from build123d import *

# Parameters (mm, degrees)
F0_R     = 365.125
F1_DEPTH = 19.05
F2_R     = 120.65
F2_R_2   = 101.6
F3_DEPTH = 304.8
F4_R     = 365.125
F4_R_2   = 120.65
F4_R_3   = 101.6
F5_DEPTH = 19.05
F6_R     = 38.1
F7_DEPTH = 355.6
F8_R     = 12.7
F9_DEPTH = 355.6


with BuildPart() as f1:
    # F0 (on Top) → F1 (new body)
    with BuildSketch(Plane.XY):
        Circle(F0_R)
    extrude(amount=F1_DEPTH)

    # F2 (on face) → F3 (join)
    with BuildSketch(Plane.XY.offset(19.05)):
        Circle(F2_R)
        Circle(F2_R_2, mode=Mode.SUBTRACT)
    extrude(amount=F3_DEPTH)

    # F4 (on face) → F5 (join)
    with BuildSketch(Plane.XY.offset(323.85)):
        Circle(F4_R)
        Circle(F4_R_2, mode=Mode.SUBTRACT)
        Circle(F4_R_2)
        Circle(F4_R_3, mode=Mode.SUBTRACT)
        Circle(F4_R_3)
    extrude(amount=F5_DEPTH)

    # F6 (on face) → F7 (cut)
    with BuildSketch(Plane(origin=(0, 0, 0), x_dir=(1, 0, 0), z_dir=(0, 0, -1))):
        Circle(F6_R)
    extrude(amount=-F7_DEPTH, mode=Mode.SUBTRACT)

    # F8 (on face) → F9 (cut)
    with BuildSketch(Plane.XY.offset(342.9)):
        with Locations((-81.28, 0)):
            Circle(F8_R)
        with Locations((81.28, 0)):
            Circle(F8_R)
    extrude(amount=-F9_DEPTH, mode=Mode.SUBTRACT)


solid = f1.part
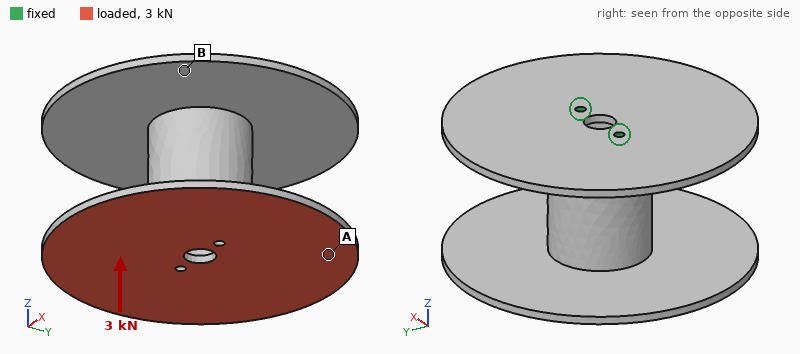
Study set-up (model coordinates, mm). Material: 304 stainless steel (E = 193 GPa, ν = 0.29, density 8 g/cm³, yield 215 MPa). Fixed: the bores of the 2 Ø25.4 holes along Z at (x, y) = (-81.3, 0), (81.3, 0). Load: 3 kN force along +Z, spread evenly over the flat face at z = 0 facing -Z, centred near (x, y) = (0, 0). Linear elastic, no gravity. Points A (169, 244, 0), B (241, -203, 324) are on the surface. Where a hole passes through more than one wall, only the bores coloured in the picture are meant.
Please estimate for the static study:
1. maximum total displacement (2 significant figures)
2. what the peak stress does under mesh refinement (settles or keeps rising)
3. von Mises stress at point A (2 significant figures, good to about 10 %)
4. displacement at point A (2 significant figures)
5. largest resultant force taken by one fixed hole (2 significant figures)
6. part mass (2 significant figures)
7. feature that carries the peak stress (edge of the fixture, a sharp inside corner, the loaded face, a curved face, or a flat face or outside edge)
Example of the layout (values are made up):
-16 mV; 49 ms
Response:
39 µm; keeps rising; 1.1 MPa; 27 µm; 1.5 kN; 160 kg; edge of the fixture
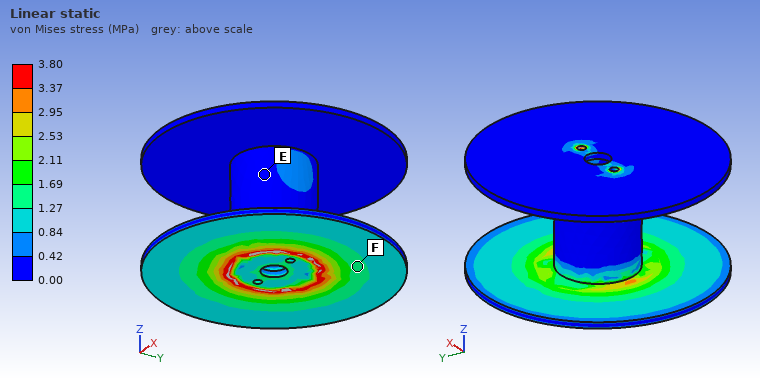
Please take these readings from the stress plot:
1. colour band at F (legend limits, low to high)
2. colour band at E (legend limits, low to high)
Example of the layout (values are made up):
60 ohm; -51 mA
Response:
1.27 to 1.69 MPa; 0.00 to 0.42 MPa
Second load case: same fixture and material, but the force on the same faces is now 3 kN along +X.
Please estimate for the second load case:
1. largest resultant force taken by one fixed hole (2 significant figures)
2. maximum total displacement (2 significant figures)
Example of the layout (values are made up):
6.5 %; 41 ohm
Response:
5.3 kN; 22 µm
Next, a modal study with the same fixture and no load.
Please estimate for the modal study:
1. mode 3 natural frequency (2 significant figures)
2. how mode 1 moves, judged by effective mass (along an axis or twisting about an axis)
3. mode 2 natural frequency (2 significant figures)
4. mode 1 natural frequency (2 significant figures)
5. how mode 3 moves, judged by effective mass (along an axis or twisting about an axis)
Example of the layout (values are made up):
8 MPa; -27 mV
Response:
210 Hz; along Y; 180 Hz; 71 Hz; along Z
